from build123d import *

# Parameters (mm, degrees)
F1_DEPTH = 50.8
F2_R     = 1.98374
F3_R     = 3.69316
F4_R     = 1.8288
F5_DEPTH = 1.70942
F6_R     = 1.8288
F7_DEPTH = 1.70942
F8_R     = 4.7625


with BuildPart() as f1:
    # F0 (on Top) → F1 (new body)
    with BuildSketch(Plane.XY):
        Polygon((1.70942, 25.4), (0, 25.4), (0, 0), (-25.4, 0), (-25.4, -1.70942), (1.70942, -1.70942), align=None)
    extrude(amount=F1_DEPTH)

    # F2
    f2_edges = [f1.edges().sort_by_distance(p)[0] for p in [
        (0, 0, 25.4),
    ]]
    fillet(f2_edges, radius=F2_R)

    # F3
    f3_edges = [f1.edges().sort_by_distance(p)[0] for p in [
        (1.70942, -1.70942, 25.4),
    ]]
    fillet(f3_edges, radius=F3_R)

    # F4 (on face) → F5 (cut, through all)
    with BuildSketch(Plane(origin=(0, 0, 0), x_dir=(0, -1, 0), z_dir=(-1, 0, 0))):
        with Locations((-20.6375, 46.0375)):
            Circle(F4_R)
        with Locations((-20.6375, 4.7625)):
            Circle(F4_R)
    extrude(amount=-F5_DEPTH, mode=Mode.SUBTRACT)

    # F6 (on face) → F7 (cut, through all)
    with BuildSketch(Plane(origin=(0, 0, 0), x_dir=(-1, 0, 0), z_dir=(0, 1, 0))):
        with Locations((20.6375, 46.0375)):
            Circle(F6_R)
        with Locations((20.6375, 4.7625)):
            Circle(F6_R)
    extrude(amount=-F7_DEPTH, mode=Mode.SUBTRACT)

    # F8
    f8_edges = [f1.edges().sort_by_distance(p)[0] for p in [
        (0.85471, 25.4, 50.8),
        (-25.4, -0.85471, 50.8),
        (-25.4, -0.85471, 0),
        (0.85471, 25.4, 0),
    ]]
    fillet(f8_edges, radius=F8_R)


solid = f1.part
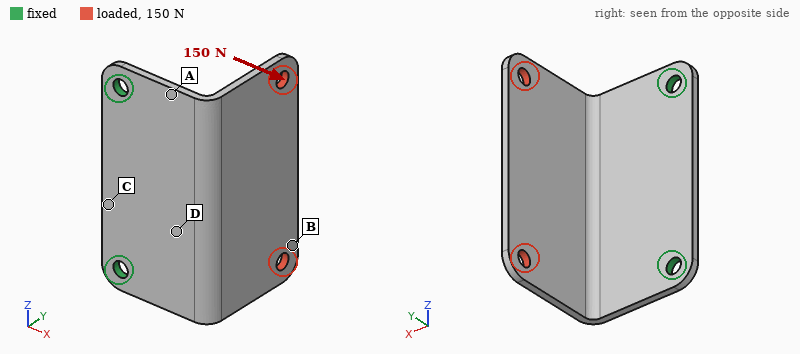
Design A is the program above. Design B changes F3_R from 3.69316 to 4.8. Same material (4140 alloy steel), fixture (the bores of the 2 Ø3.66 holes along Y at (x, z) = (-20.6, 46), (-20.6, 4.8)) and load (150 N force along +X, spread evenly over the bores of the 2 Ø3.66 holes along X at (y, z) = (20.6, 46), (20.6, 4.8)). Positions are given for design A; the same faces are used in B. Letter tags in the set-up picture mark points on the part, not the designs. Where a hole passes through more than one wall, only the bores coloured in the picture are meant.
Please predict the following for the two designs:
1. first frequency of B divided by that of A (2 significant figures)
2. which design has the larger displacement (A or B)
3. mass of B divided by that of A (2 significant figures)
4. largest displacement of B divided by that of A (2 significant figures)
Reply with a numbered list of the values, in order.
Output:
1. 0.98
2. B
3. 0.98
4. 1.1
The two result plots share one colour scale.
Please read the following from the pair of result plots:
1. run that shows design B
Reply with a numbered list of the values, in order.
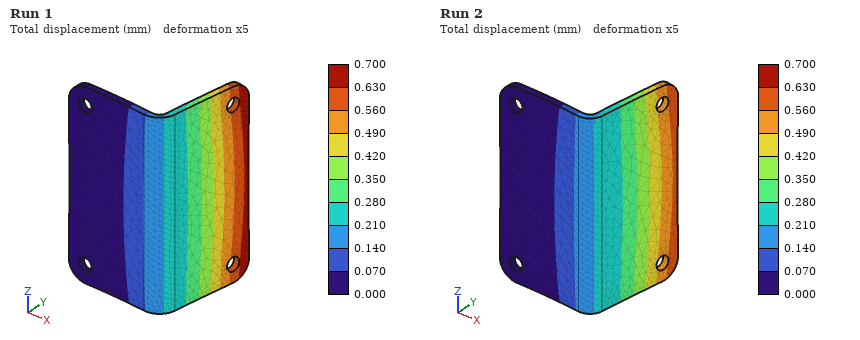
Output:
1. Run 1
